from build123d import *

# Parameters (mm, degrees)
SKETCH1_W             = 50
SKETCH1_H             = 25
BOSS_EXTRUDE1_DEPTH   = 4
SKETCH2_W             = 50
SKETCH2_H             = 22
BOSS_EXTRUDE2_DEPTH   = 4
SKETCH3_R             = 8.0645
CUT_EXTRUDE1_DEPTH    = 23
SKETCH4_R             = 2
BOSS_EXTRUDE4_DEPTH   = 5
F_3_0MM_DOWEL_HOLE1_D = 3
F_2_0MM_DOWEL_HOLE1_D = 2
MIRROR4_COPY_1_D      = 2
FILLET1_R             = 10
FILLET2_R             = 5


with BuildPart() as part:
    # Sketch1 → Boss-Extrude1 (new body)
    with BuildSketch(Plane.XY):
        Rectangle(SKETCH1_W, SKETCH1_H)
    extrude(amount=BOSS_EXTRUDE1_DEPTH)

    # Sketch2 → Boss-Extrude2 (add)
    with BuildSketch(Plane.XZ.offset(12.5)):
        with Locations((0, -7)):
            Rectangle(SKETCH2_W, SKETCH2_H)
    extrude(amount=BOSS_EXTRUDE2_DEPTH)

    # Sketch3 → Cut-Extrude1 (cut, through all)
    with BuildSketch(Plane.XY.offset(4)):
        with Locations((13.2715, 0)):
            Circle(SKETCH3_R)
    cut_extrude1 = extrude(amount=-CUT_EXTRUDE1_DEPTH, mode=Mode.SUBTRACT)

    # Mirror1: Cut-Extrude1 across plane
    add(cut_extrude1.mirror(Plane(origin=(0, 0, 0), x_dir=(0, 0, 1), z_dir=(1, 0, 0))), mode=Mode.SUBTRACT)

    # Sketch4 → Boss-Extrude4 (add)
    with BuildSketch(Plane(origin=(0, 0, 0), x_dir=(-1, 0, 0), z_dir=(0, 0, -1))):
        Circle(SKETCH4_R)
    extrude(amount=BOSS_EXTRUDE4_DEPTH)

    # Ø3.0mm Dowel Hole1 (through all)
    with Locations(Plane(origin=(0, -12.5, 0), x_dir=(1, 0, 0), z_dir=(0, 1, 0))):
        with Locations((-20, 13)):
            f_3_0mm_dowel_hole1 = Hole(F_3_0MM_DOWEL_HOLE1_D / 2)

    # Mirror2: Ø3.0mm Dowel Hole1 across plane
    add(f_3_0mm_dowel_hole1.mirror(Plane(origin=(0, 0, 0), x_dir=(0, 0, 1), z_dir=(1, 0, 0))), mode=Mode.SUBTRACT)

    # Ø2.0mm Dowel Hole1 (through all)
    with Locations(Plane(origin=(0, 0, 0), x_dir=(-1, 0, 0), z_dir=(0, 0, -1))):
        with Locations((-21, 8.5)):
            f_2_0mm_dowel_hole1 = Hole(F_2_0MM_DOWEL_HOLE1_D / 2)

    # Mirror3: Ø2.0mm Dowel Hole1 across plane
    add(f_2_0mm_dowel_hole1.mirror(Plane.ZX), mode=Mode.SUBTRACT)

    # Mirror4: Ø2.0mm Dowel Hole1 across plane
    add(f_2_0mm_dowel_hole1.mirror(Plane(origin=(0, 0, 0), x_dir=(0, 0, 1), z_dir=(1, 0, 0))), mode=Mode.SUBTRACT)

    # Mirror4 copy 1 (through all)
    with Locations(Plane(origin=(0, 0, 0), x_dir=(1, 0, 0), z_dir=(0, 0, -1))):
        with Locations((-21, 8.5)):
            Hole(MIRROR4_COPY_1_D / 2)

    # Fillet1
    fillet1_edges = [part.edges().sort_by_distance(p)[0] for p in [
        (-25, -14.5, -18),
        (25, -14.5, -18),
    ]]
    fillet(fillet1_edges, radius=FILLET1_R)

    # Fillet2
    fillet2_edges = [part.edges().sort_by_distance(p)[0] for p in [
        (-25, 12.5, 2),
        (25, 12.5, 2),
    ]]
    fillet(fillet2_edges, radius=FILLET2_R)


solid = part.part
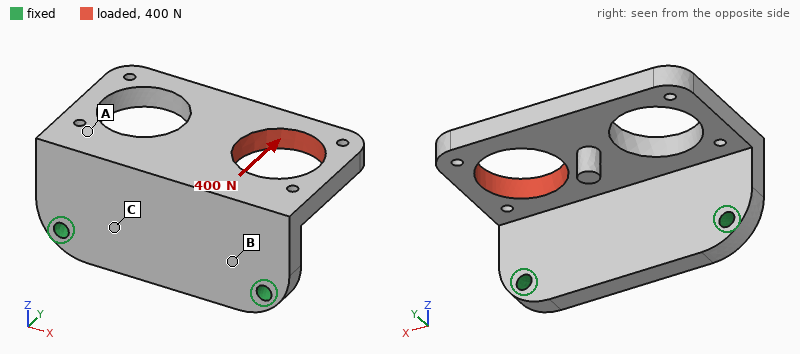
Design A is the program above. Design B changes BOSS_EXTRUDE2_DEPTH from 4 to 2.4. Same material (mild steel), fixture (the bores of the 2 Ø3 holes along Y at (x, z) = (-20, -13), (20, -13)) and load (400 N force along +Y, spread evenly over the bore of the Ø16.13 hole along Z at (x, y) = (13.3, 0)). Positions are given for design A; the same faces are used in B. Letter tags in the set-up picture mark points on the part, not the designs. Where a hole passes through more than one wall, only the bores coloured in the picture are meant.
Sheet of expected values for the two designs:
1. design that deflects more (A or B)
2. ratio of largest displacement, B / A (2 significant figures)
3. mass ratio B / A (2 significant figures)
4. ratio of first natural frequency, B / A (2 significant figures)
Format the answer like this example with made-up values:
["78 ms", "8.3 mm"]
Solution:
["B", "3.6", "0.78", "0.57"]
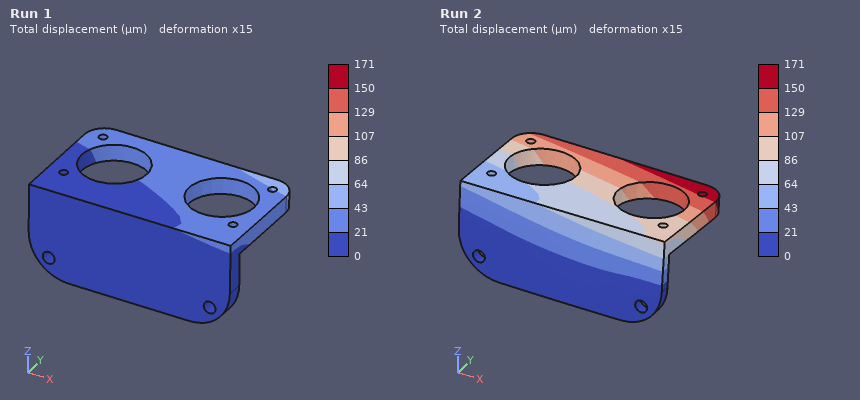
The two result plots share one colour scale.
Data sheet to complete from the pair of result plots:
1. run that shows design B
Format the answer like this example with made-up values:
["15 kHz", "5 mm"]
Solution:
["Run 2"]
